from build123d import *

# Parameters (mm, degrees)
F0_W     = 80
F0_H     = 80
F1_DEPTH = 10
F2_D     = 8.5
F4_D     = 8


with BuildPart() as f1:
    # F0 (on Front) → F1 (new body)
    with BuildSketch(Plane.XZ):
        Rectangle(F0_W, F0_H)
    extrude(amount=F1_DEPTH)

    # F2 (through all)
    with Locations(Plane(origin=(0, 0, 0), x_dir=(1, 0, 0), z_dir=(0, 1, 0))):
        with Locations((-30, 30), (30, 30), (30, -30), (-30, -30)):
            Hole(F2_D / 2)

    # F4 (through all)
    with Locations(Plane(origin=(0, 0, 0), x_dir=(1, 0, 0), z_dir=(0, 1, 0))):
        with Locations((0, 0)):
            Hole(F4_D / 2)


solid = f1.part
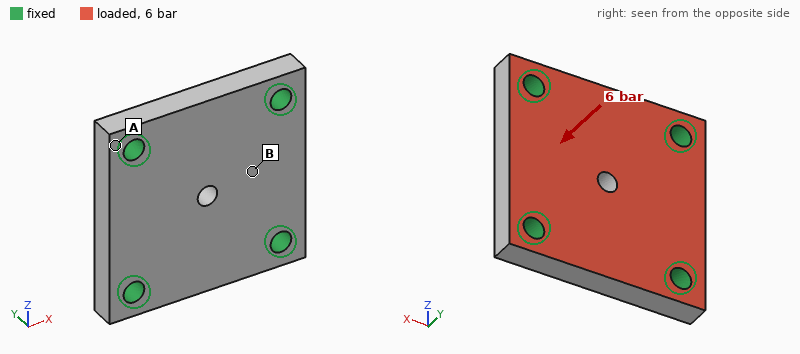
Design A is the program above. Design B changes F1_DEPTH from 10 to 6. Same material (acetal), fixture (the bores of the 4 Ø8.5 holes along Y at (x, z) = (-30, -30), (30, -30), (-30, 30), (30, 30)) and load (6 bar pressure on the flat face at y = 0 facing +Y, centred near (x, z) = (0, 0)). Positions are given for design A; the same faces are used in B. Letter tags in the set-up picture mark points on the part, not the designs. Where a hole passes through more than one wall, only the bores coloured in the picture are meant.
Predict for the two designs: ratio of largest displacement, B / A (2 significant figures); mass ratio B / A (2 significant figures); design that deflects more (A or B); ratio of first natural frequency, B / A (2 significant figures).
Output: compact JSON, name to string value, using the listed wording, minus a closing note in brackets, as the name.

{"ratio of largest displacement, B / A": "3.7", "mass ratio B / A": "0.60", "design that deflects more": "B", "ratio of first natural frequency, B / A": "0.68"}
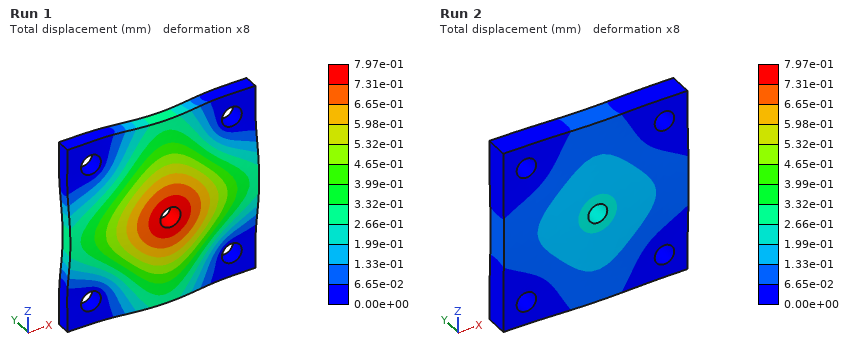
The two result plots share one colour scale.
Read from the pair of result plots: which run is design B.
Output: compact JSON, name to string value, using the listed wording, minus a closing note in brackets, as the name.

{"which run is design B": "Run 1"}
